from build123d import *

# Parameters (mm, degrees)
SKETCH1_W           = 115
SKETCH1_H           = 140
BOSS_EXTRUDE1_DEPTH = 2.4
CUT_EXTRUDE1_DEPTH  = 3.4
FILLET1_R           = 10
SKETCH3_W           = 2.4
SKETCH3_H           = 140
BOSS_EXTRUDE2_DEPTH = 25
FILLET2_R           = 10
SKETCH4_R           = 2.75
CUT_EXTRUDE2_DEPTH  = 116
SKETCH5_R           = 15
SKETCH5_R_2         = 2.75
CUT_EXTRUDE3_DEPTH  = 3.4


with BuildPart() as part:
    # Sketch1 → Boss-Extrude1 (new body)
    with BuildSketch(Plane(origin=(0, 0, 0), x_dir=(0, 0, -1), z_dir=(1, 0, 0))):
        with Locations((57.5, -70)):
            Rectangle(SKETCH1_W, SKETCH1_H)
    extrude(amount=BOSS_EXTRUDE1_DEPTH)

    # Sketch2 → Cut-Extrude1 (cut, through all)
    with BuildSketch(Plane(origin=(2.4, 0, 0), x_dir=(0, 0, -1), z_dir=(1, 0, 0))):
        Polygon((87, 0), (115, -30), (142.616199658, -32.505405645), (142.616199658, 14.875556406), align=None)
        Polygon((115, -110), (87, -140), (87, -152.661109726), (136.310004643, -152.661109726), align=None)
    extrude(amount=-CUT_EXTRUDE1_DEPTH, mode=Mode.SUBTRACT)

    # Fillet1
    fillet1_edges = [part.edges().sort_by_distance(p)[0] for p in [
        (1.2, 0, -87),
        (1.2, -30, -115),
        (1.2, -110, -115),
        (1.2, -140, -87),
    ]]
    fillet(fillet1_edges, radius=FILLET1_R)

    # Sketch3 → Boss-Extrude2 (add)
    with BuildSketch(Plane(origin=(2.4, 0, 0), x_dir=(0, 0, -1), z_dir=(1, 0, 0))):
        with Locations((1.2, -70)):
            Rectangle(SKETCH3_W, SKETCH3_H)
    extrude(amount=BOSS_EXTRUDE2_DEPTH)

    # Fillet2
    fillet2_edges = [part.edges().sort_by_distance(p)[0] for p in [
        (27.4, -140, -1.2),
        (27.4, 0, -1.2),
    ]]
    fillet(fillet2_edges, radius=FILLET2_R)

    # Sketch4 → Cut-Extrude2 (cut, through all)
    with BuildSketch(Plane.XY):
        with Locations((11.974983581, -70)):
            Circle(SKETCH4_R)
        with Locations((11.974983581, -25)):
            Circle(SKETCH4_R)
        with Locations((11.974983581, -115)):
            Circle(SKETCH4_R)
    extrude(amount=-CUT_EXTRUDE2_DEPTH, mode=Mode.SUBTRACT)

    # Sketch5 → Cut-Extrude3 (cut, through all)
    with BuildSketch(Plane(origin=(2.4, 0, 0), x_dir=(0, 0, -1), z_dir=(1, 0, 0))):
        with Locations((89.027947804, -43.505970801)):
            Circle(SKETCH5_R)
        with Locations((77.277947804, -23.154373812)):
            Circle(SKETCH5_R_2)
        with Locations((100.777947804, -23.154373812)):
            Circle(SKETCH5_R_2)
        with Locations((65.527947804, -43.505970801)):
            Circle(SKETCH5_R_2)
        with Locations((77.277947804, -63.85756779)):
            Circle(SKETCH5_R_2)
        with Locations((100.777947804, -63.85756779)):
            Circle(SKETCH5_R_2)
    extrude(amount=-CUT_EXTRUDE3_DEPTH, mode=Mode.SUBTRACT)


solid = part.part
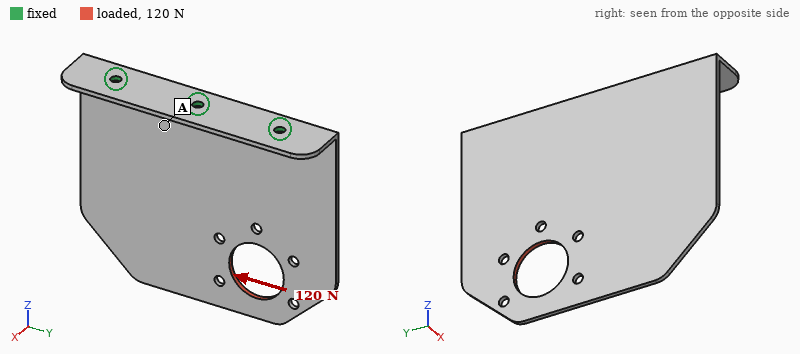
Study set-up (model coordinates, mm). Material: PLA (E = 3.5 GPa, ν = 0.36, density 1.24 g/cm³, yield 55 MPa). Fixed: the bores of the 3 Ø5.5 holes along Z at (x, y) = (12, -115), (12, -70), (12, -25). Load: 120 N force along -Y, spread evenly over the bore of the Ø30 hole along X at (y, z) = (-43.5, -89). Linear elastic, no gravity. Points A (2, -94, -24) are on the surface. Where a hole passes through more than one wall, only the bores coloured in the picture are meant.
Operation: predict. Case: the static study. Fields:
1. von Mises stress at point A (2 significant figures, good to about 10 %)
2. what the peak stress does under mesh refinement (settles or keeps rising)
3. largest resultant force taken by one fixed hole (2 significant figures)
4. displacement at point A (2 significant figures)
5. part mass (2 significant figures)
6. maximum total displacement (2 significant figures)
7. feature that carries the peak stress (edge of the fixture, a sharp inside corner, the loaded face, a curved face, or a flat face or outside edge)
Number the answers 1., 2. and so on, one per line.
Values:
1. 2.8 MPa
2. keeps rising
3. 120 N
4. 0.31 mm
5. 53 g
6. 1.4 mm
7. edge of the fixture
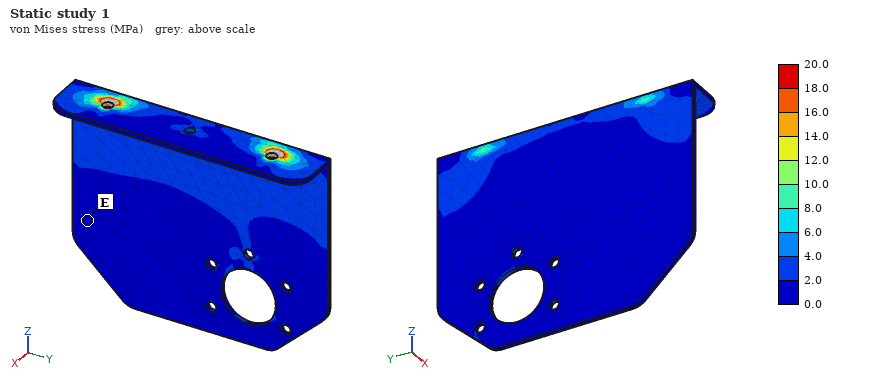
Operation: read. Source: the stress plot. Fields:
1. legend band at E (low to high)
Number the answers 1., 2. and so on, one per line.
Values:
1. 0.0 to 2.0 MPa
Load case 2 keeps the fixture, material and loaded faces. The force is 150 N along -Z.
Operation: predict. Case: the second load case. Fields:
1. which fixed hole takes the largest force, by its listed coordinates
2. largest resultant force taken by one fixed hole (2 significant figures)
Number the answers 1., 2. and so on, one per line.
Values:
1. (12, -25)
2. 93 N
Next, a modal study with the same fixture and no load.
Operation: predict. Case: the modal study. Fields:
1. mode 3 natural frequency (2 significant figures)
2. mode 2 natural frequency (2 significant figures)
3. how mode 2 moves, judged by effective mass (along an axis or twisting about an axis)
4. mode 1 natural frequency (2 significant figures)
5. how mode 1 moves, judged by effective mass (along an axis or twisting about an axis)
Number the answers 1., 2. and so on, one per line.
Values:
1. 260 Hz
2. 120 Hz
3. twisting about Z
4. 52 Hz
5. along X
